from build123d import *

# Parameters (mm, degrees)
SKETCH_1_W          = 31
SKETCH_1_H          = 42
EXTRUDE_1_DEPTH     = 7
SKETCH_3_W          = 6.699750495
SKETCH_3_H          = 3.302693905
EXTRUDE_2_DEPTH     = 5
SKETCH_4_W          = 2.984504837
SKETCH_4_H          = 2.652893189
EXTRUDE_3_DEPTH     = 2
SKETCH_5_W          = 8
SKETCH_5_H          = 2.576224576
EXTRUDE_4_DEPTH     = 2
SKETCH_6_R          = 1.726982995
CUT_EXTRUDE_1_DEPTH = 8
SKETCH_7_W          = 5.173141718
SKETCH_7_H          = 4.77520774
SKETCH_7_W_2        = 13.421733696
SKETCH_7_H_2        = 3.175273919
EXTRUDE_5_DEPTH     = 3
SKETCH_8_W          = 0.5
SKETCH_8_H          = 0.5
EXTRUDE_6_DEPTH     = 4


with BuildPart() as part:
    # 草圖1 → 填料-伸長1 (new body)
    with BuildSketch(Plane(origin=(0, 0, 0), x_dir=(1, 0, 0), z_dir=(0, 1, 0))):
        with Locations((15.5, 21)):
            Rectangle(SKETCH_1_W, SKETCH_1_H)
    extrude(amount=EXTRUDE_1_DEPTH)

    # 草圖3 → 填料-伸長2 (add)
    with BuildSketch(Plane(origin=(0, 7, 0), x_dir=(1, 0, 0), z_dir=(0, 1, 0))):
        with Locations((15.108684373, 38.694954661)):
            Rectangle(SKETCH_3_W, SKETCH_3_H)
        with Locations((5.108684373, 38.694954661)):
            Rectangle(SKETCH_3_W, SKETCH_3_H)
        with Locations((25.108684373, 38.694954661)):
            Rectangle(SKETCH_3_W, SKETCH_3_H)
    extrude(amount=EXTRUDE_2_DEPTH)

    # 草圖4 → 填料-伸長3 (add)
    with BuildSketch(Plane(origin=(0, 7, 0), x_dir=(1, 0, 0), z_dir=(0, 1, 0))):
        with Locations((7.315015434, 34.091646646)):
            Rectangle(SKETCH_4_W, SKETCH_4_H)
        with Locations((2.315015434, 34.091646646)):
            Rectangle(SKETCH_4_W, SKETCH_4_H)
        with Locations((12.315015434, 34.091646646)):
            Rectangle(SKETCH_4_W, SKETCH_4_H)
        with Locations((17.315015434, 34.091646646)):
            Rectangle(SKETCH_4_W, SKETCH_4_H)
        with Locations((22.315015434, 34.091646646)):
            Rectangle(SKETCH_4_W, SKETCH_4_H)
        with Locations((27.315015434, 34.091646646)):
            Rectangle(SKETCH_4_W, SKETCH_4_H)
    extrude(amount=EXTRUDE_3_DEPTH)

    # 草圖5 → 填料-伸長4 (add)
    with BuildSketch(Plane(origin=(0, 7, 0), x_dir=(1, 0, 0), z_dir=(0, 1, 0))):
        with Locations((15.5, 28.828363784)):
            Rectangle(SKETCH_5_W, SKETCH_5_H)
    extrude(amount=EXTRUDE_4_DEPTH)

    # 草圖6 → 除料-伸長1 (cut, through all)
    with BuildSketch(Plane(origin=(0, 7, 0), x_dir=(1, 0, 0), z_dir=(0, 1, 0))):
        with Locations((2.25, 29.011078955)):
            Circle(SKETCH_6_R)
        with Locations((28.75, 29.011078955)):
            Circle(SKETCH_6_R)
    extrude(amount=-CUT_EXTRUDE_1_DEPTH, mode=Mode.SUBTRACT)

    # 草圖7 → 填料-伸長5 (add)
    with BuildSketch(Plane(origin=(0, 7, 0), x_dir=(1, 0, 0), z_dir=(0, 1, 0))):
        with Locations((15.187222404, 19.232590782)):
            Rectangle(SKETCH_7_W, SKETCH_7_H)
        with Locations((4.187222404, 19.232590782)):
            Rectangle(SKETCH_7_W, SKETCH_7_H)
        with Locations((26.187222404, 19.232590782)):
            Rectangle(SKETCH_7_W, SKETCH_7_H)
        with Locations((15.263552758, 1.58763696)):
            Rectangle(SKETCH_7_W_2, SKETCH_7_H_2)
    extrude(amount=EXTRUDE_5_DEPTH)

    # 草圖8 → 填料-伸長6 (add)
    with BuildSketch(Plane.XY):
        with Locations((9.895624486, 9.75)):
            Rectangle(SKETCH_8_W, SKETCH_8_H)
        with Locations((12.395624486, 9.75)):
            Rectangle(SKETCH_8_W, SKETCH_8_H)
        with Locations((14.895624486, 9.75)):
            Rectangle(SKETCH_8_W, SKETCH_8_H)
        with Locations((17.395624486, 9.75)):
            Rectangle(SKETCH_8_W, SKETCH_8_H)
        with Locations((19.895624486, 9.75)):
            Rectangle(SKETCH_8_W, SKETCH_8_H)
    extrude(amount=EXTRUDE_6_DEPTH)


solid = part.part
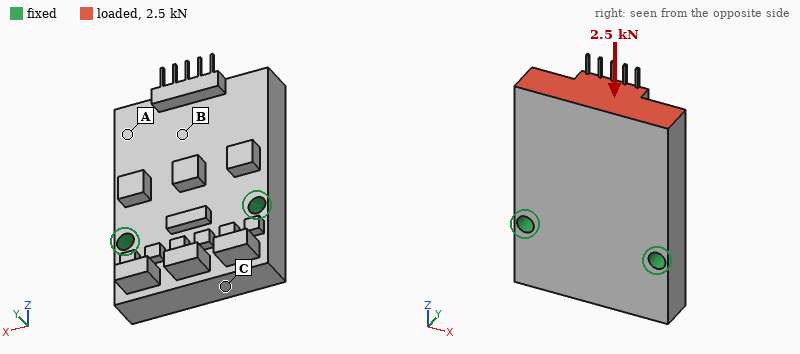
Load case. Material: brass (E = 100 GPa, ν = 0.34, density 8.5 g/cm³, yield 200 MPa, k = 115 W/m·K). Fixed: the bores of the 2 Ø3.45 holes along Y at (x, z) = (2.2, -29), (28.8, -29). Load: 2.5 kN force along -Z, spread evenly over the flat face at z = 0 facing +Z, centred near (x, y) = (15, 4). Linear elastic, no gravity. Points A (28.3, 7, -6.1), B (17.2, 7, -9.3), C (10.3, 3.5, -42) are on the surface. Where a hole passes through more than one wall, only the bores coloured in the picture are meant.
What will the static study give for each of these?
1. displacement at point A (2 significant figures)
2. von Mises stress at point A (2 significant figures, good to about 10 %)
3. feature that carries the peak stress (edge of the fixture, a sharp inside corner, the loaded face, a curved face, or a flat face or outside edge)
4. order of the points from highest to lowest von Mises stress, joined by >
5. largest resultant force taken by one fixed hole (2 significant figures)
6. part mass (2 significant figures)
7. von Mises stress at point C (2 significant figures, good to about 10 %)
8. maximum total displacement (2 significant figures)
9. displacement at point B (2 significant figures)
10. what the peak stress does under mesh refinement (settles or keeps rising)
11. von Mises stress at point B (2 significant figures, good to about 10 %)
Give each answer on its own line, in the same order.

7.5 µm
14 MPa
edge of the fixture
B > A > C
1.3 kN
83 g
5.7 MPa
18 µm
6.7 µm
keeps rising
21 MPa
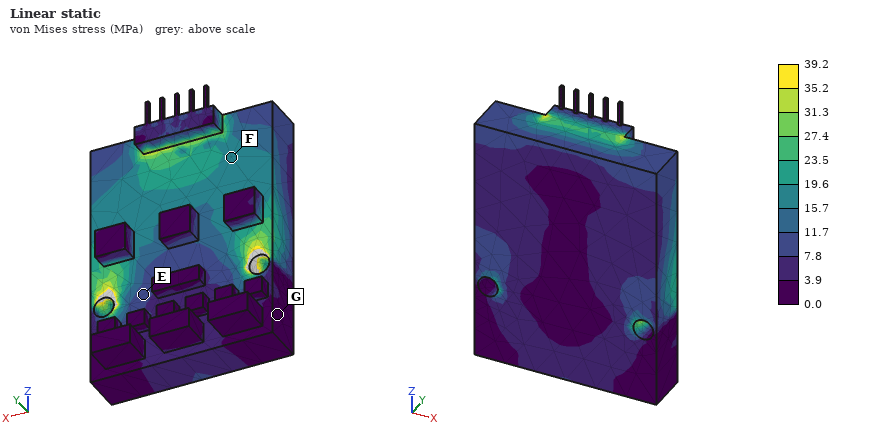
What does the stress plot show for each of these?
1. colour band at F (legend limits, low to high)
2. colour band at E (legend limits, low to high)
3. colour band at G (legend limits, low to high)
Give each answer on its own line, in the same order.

15.7 to 19.6 MPa
7.8 to 11.7 MPa
0.0 to 3.9 MPa
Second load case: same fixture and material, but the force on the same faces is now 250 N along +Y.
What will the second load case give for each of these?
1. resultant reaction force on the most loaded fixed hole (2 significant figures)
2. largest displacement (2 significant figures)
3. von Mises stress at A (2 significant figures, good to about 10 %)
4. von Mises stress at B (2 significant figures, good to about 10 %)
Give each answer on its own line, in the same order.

130 N
35 µm
6.1 MPa
9.9 MPa
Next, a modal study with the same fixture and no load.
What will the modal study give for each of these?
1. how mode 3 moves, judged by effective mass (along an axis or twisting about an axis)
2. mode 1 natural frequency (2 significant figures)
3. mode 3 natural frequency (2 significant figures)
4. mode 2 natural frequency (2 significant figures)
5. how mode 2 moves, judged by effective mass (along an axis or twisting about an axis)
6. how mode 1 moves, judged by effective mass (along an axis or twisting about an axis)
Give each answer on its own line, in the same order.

along X
3800 Hz
13 kHz
9400 Hz
twisting about Z
along Y
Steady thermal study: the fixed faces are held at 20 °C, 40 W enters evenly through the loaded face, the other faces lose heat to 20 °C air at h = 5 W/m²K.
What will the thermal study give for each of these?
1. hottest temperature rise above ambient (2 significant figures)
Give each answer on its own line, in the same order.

53 K
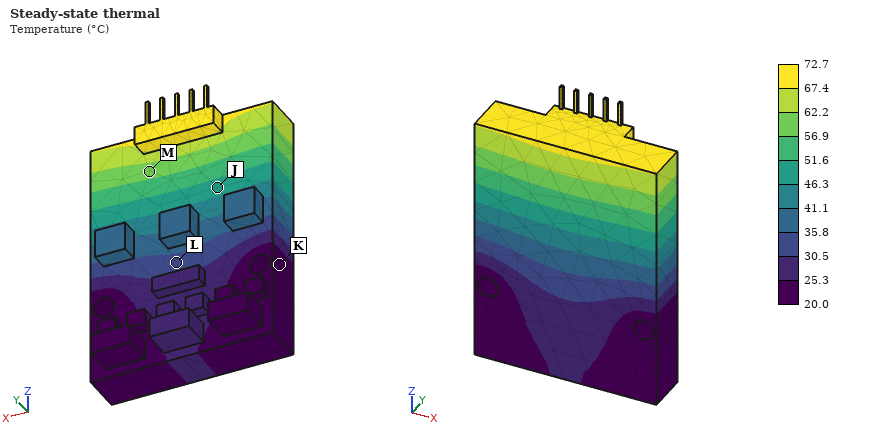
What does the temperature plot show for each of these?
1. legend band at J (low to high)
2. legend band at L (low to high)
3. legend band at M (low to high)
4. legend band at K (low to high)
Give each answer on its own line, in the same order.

46.3 to 51.6 °C
30.5 to 35.8 °C
56.9 to 62.2 °C
20.0 to 25.3 °C
